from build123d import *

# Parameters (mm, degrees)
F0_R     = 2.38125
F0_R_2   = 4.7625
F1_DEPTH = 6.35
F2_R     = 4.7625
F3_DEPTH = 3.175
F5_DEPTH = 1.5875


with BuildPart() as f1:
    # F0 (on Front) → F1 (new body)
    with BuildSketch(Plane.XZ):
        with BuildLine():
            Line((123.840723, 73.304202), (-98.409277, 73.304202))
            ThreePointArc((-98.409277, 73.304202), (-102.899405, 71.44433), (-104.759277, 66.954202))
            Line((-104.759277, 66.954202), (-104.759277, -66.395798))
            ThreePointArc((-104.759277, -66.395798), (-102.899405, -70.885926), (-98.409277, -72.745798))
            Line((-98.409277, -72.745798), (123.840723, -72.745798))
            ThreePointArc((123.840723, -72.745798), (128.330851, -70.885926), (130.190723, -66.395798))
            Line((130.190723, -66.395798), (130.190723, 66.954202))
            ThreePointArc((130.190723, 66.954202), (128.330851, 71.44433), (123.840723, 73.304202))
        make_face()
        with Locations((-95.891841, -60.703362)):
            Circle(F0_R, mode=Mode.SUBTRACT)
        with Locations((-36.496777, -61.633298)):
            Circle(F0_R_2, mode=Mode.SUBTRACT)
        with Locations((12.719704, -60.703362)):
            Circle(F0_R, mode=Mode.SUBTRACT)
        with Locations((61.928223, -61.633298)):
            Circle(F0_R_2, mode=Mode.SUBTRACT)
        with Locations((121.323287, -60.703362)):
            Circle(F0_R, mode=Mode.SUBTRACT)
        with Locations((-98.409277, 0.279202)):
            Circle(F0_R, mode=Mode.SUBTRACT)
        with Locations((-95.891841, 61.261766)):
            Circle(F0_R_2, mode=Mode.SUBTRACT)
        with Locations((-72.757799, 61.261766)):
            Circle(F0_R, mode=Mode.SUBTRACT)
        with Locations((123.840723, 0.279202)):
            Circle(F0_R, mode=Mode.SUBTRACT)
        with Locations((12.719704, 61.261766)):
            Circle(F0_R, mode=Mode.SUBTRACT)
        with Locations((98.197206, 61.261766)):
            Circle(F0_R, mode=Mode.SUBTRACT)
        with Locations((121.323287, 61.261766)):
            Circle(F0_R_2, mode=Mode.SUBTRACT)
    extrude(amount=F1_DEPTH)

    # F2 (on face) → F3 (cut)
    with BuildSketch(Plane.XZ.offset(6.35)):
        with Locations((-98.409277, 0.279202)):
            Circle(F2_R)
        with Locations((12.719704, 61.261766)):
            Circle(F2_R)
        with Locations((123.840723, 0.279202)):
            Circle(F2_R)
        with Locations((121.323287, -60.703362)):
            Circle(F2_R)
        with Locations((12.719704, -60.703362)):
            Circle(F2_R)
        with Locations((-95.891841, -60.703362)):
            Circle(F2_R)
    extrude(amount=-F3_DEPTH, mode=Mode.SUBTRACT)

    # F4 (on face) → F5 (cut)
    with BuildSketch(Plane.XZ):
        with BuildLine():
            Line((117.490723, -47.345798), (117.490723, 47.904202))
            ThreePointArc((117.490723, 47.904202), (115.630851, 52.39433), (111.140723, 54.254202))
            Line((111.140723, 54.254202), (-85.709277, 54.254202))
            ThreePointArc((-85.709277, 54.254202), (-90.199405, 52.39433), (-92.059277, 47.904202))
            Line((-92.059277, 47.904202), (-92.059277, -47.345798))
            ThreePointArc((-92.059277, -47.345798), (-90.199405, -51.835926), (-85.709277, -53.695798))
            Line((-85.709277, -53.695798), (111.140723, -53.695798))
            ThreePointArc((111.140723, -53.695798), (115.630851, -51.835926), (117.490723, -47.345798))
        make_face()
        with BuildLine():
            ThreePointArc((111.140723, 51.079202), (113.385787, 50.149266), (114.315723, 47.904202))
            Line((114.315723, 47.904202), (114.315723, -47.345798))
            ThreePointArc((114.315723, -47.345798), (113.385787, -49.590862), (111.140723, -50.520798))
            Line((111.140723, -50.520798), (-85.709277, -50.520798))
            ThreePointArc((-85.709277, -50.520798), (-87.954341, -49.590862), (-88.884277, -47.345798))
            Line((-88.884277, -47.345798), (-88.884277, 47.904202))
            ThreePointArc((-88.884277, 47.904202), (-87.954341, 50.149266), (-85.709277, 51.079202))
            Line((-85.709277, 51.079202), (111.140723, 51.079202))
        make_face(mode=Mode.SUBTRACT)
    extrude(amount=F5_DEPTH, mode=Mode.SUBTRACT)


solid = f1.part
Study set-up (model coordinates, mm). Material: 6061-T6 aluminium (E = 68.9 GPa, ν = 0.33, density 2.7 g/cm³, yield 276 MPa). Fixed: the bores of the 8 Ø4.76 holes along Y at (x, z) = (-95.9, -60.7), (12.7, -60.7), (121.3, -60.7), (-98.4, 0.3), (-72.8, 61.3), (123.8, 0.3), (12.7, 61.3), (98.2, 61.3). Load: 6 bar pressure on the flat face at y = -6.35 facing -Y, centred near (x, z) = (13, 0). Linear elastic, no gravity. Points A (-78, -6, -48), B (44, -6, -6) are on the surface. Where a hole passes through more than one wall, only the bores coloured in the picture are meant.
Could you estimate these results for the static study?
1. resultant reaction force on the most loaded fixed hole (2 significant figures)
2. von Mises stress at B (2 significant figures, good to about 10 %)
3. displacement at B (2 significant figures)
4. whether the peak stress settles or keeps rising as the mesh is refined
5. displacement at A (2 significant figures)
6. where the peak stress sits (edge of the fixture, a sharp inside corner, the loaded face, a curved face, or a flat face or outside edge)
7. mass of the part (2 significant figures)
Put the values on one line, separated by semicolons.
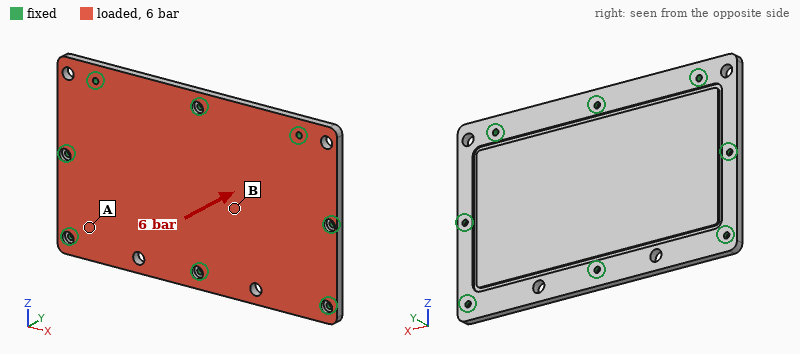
5.7 kN; 74 MPa; 0.52 mm; keeps rising; 0.16 mm; edge of the fixture; 570 g
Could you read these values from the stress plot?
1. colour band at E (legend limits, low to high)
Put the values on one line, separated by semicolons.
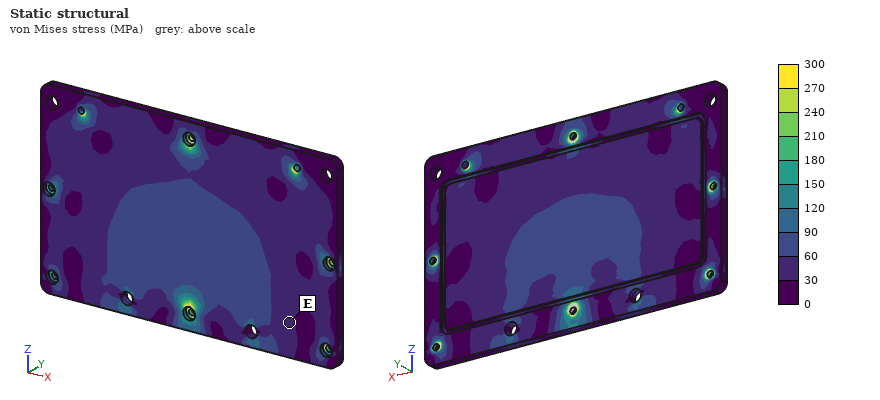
30 to 60 MPa
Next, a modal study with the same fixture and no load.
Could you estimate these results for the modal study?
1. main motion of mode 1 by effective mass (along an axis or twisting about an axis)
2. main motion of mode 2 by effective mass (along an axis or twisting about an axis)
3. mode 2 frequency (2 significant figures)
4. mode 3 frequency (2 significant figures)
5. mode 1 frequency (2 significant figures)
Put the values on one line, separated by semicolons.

along Y; twisting about Z; 1900 Hz; 2700 Hz; 1500 Hz
